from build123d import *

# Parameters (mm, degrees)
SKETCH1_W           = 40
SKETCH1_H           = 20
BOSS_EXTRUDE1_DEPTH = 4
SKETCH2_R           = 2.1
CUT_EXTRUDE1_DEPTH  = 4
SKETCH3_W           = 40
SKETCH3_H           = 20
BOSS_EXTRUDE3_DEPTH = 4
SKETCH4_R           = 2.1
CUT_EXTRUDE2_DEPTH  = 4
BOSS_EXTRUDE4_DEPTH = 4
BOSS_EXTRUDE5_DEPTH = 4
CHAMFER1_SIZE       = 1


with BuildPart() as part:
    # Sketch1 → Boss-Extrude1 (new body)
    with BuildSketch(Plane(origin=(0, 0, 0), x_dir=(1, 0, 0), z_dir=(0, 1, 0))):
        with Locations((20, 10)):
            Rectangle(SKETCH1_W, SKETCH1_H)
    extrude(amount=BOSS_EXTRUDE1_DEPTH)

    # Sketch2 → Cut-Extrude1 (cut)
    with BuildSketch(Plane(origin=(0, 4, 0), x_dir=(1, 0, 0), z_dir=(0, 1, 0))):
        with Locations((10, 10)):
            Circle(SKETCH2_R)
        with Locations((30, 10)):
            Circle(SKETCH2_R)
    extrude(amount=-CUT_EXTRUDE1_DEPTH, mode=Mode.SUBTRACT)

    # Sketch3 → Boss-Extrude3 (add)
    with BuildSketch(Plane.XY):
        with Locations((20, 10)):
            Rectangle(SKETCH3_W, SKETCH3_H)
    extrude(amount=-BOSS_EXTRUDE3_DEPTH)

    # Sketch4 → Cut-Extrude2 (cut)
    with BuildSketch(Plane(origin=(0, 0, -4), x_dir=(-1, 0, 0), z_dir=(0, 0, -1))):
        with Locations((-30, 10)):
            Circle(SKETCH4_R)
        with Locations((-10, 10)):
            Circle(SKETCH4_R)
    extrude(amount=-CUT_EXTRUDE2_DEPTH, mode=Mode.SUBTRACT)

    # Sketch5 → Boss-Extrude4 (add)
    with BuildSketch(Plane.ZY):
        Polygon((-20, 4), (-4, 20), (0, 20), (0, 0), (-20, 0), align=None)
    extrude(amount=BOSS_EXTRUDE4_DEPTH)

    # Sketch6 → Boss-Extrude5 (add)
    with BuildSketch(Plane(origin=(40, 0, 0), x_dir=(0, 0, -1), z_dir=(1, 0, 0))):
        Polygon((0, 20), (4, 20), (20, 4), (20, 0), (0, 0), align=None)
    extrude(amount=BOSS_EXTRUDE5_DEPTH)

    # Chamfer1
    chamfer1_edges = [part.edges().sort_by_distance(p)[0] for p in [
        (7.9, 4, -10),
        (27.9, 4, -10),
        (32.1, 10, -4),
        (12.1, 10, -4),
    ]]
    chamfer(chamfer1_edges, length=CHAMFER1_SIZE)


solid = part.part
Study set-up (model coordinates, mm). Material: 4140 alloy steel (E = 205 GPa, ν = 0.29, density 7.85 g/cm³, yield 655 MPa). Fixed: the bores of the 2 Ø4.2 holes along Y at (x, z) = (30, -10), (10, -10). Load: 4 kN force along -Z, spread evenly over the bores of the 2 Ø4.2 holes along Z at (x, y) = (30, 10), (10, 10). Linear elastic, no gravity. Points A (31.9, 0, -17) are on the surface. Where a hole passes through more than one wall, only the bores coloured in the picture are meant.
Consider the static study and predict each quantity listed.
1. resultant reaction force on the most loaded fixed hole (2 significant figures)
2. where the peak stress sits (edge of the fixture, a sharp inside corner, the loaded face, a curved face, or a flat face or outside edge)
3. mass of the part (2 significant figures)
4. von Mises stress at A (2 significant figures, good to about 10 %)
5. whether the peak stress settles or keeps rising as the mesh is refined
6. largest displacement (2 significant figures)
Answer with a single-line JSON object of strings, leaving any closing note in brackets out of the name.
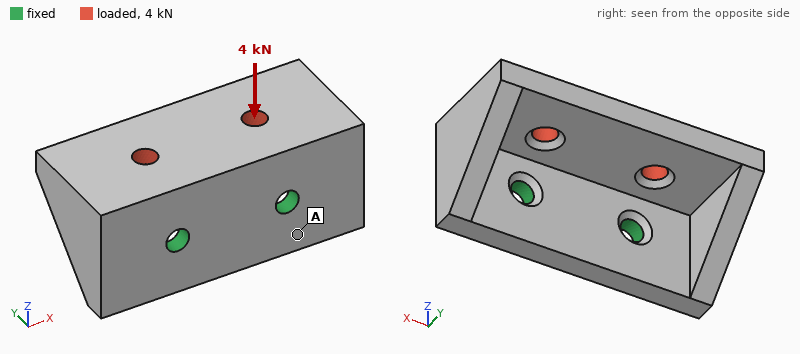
{"resultant reaction force on the most loaded fixed hole": "2.0 kN", "where the peak stress sits": "edge of the fixture", "mass of the part": "60 g", "von Mises stress at A": "97 MPa", "whether the peak stress settles or keeps rising as the mesh is refined": "keeps rising", "largest displacement": "0.11 mm"}
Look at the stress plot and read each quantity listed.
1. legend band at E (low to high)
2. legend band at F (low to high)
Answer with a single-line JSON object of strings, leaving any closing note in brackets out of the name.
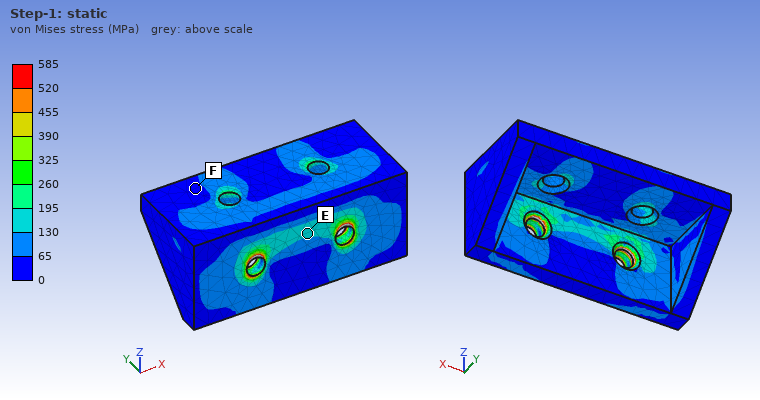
{"legend band at E": "130 to 195 MPa", "legend band at F": "0 to 65 MPa"}
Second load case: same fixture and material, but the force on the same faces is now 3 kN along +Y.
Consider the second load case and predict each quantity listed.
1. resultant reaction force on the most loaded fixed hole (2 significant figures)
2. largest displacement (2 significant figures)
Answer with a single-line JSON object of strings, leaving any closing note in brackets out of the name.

{"resultant reaction force on the most loaded fixed hole": "1.5 kN", "largest displacement": "51 µm"}
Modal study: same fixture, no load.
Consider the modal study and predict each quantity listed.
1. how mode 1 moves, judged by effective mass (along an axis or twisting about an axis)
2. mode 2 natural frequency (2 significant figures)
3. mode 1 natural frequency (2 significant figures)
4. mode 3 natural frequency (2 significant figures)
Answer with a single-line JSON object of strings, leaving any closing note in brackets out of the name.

{"how mode 1 moves, judged by effective mass": "along Z", "mode 2 natural frequency": "7500 Hz", "mode 1 natural frequency": "6100 Hz", "mode 3 natural frequency": "12 kHz"}
